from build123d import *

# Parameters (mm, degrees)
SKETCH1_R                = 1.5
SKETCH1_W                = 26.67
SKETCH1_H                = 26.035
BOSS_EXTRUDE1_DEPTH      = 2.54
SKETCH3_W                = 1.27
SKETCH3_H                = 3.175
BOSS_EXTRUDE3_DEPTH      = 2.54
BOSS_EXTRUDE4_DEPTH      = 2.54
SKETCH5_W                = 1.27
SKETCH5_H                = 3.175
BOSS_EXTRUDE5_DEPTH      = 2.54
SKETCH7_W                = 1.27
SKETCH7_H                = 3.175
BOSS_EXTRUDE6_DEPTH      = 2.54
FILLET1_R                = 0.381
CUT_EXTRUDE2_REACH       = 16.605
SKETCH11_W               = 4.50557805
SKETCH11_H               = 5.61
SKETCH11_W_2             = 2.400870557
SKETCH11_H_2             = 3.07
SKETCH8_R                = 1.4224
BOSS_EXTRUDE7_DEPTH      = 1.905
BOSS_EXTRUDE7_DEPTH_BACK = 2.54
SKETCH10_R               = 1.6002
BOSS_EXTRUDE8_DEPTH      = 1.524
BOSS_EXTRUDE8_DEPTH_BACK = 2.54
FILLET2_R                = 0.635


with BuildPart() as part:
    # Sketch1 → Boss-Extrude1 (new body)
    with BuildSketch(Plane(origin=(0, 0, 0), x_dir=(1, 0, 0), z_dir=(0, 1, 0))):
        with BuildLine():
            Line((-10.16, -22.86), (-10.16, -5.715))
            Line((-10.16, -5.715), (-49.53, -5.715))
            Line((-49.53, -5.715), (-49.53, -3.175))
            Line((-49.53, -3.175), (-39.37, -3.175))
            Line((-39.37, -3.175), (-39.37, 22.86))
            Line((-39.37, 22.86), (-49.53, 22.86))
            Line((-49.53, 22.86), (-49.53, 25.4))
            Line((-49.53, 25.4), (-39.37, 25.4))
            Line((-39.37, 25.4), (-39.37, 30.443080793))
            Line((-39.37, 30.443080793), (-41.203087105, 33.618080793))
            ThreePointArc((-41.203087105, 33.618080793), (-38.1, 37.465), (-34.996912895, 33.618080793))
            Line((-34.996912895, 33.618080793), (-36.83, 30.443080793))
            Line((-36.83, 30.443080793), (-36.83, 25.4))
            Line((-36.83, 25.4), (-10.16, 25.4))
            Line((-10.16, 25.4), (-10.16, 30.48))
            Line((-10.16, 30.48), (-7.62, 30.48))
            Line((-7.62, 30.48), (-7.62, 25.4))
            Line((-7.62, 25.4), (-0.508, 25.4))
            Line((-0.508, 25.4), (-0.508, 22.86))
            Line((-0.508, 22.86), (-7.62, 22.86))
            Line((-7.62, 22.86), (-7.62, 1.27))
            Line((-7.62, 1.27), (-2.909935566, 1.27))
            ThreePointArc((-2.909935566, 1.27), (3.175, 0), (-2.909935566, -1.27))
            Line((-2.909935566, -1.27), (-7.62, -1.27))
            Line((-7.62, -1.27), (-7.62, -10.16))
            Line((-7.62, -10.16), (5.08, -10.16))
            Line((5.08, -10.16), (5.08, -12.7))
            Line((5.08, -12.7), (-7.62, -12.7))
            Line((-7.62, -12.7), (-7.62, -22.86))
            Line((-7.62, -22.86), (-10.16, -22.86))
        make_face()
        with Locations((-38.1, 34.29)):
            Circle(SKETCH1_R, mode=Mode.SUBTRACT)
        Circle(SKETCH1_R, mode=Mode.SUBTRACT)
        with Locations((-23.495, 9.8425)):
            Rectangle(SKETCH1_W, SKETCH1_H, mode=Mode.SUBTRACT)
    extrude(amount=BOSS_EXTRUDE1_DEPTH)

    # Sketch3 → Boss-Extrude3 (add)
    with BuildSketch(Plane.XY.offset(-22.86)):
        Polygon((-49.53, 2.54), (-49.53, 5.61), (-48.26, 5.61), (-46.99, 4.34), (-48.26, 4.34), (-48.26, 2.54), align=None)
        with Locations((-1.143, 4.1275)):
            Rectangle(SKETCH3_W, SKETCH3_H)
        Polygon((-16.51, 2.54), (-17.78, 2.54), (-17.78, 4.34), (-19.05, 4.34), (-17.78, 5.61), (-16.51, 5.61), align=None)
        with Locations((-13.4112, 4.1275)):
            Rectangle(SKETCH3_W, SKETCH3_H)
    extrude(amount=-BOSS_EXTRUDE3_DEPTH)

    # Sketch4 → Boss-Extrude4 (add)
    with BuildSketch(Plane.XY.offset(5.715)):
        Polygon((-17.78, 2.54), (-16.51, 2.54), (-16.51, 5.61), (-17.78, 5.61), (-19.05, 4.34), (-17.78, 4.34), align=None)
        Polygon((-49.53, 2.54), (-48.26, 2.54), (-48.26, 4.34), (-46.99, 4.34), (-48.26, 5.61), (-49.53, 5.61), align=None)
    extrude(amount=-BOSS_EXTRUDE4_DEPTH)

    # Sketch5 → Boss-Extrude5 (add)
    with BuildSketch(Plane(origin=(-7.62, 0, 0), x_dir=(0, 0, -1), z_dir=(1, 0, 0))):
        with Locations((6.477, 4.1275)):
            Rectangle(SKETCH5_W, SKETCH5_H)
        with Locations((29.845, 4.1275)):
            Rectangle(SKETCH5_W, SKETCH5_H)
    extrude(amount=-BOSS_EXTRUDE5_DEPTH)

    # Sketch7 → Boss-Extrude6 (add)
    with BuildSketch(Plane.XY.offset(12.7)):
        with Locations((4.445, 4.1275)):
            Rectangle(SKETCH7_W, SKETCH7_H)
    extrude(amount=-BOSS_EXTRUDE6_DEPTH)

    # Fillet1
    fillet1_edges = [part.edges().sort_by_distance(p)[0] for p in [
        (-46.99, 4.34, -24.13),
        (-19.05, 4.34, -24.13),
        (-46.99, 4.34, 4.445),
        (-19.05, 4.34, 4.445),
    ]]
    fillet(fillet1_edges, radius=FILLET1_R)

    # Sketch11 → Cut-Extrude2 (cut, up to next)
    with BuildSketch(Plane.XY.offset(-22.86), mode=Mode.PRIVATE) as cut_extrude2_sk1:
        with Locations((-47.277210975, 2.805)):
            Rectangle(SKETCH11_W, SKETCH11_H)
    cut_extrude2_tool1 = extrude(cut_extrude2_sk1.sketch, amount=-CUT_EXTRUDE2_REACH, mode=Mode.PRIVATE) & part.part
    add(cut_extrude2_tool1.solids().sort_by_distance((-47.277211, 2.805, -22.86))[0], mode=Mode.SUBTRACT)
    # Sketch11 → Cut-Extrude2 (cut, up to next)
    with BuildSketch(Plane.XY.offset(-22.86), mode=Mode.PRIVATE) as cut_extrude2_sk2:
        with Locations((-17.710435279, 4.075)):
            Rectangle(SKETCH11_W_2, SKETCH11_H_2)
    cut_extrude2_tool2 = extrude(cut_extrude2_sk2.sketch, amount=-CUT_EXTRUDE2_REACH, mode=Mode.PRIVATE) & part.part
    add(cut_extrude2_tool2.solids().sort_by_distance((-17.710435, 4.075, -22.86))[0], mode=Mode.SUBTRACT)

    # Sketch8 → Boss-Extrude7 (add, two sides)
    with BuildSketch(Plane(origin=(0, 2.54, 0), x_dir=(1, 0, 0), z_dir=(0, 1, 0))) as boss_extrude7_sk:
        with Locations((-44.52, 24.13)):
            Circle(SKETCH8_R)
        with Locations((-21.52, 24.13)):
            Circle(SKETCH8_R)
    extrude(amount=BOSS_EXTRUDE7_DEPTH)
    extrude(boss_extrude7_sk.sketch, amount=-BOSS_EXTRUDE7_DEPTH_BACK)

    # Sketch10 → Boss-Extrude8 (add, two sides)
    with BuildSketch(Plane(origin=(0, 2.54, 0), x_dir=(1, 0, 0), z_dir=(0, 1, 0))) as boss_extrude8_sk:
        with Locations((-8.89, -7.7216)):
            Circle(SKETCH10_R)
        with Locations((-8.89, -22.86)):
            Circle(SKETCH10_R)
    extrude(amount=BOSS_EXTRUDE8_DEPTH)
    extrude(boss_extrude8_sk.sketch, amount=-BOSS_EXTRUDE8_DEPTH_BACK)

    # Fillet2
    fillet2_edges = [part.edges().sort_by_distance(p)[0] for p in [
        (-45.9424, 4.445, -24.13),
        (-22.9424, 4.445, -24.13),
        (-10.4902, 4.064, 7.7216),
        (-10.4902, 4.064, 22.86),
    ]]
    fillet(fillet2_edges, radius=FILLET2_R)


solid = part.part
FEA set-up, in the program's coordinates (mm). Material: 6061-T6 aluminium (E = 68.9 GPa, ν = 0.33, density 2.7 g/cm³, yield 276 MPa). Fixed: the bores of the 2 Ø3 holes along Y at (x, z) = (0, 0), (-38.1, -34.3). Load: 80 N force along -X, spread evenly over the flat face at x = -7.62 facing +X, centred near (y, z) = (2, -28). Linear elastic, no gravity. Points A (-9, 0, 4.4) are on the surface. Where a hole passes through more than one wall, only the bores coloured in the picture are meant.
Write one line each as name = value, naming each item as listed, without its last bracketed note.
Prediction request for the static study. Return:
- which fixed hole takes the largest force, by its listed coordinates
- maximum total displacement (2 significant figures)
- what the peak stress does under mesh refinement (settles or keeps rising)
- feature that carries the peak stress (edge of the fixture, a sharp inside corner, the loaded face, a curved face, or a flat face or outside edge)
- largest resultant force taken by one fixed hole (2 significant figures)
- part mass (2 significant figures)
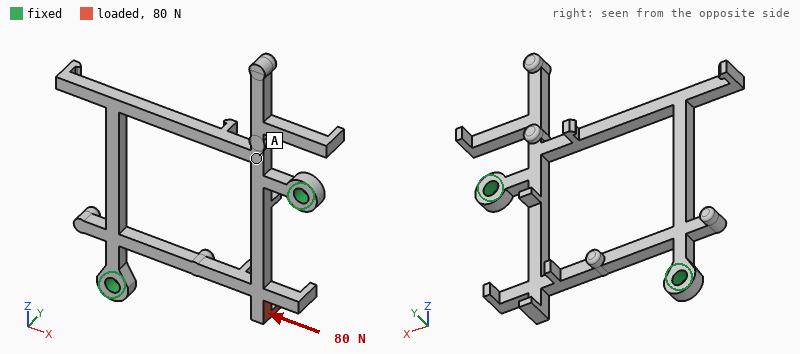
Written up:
which fixed hole takes the largest force, by its listed coordinates = (-38.1, -34.3)
maximum total displacement = 0.12 mm
what the peak stress does under mesh refinement = keeps rising
feature that carries the peak stress = a sharp inside corner
largest resultant force taken by one fixed hole = 81 N
part mass = 3.9 g
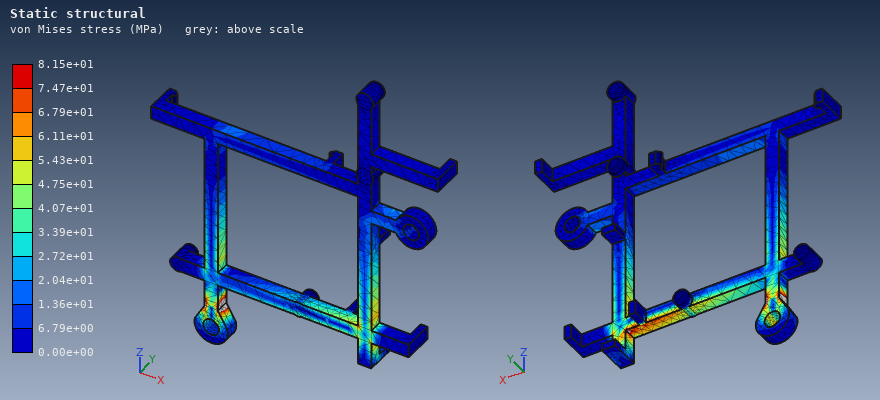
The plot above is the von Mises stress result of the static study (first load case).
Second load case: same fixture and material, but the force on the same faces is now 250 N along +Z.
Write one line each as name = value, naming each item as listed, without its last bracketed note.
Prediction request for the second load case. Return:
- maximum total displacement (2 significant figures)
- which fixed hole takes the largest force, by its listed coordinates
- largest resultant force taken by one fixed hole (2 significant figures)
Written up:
maximum total displacement = 0.28 mm
which fixed hole takes the largest force, by its listed coordinates = (0, 0)
largest resultant force taken by one fixed hole = 240 N
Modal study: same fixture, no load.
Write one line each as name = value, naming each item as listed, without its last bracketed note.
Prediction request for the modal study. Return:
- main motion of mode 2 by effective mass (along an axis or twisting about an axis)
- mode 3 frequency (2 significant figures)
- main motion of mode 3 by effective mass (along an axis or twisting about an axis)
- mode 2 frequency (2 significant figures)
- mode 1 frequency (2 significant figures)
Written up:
main motion of mode 2 by effective mass = along Y
mode 3 frequency = 2400 Hz
main motion of mode 3 by effective mass = along Y
mode 2 frequency = 1600 Hz
mode 1 frequency = 1100 Hz
